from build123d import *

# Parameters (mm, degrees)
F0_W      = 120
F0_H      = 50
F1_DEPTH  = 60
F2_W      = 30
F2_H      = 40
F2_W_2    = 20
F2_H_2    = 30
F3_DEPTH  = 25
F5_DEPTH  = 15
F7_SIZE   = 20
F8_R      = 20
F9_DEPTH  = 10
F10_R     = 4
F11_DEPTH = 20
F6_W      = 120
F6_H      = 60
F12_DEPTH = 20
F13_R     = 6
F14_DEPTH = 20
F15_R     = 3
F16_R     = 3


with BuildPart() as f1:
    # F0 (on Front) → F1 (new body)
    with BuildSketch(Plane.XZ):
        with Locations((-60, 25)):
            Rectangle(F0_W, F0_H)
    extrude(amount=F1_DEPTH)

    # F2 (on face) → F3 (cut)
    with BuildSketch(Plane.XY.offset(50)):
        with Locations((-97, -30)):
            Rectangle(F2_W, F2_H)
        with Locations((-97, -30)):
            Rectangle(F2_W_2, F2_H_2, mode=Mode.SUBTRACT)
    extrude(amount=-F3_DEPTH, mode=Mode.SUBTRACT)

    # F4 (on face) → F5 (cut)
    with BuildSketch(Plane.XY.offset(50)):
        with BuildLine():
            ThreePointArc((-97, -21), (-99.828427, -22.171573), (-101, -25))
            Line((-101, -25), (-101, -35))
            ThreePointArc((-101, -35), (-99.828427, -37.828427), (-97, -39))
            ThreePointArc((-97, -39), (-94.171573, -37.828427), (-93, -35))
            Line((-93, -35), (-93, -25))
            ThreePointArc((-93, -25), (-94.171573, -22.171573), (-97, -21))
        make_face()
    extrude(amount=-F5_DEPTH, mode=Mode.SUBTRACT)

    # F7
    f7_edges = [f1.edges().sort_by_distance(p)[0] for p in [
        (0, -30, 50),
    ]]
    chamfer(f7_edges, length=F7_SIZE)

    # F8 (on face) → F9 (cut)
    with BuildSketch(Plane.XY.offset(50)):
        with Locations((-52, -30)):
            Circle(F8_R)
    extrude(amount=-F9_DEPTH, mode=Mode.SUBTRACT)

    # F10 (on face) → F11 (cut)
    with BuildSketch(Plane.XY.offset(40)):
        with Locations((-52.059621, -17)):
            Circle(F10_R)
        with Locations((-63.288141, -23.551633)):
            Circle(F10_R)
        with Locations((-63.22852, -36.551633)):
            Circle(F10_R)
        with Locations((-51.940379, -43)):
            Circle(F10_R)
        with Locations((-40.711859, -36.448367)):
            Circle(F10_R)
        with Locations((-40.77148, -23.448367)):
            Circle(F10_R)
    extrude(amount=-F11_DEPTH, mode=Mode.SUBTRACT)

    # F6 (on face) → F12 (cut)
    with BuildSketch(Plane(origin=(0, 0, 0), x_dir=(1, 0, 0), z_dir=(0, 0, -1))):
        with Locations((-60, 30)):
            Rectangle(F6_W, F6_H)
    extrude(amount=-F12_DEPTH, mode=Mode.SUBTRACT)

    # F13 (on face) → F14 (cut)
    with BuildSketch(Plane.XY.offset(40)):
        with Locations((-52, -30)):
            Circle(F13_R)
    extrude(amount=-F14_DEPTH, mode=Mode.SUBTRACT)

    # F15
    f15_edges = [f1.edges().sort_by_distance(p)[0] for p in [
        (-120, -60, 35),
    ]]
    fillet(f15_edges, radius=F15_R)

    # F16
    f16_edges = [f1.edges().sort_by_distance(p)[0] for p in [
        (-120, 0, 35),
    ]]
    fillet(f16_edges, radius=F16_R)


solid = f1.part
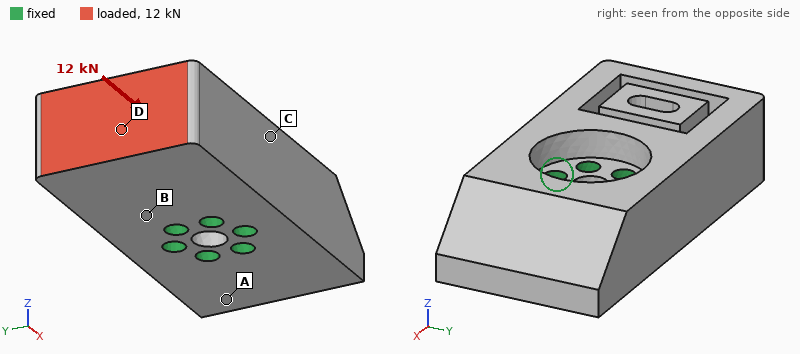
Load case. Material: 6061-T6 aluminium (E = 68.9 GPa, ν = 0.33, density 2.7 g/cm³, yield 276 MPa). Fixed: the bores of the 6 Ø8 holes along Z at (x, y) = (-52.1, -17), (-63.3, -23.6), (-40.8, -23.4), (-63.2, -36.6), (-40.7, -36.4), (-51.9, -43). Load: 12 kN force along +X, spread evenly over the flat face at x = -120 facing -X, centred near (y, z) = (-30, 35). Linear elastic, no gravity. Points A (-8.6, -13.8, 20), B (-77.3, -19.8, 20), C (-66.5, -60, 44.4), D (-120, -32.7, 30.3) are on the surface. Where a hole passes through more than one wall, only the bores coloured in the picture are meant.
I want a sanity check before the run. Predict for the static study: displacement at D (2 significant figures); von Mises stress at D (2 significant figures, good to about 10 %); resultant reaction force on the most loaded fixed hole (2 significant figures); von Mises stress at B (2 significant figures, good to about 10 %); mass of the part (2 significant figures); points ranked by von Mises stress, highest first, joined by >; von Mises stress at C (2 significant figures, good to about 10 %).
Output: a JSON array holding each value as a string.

["44 µm", "27 MPa", "2.9 kN", "13 MPa", "450 g", "D > C > B > A", "20 MPa"]
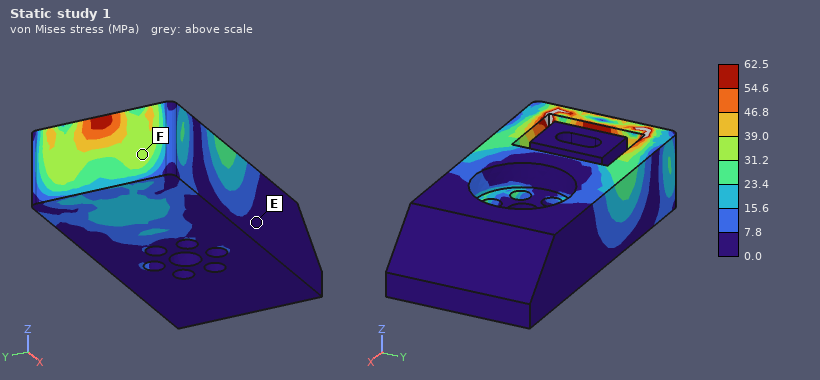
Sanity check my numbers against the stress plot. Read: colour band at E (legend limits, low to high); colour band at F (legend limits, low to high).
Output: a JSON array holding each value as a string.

["0.0 to 7.8 MPa", "31.2 to 39.0 MPa"]
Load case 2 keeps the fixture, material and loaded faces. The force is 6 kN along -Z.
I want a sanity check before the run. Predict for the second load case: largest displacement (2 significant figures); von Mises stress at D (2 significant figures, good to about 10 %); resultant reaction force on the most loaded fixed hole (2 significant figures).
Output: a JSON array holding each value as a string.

["0.15 mm", "22 MPa", "5.0 kN"]
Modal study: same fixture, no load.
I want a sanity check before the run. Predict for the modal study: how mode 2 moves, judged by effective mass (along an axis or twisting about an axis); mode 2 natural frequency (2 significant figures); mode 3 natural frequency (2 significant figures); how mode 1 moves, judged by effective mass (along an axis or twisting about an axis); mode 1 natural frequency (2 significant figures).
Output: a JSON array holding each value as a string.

["along Y", "4900 Hz", "7800 Hz", "along Z", "4200 Hz"]
